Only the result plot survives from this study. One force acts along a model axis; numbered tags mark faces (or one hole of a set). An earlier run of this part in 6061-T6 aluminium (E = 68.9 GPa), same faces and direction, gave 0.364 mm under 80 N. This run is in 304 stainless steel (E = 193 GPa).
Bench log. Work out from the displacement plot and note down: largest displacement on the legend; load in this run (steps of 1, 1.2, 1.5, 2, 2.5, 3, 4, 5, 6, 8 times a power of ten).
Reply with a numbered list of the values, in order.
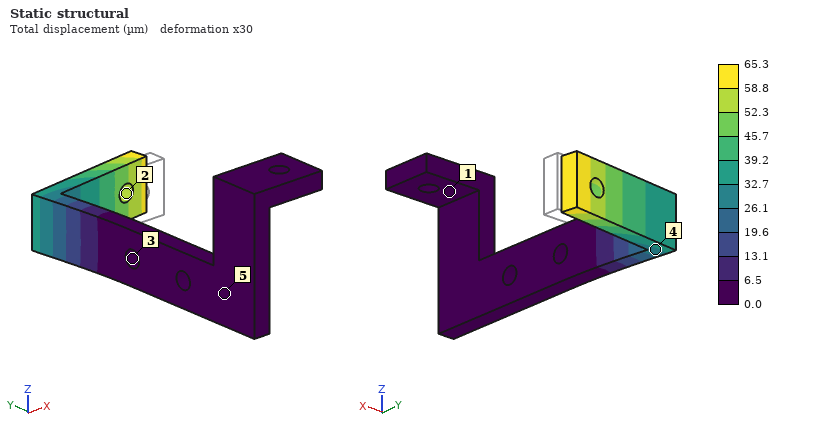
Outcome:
1. 65.3 µm
2. 40 N
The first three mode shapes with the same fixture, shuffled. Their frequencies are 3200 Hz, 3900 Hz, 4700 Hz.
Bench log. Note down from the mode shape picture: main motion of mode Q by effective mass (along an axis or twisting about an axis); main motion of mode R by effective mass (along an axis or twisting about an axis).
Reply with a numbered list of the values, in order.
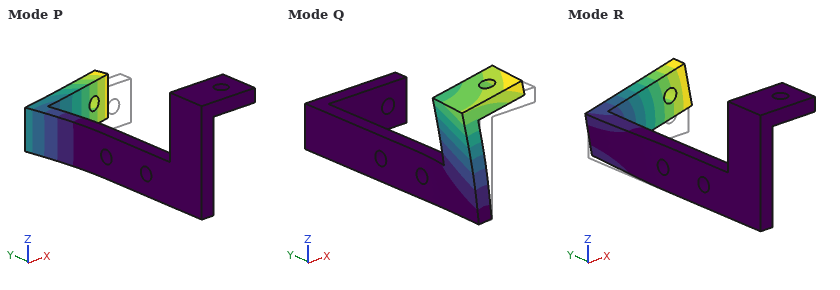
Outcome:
1. along X
2. along Z
